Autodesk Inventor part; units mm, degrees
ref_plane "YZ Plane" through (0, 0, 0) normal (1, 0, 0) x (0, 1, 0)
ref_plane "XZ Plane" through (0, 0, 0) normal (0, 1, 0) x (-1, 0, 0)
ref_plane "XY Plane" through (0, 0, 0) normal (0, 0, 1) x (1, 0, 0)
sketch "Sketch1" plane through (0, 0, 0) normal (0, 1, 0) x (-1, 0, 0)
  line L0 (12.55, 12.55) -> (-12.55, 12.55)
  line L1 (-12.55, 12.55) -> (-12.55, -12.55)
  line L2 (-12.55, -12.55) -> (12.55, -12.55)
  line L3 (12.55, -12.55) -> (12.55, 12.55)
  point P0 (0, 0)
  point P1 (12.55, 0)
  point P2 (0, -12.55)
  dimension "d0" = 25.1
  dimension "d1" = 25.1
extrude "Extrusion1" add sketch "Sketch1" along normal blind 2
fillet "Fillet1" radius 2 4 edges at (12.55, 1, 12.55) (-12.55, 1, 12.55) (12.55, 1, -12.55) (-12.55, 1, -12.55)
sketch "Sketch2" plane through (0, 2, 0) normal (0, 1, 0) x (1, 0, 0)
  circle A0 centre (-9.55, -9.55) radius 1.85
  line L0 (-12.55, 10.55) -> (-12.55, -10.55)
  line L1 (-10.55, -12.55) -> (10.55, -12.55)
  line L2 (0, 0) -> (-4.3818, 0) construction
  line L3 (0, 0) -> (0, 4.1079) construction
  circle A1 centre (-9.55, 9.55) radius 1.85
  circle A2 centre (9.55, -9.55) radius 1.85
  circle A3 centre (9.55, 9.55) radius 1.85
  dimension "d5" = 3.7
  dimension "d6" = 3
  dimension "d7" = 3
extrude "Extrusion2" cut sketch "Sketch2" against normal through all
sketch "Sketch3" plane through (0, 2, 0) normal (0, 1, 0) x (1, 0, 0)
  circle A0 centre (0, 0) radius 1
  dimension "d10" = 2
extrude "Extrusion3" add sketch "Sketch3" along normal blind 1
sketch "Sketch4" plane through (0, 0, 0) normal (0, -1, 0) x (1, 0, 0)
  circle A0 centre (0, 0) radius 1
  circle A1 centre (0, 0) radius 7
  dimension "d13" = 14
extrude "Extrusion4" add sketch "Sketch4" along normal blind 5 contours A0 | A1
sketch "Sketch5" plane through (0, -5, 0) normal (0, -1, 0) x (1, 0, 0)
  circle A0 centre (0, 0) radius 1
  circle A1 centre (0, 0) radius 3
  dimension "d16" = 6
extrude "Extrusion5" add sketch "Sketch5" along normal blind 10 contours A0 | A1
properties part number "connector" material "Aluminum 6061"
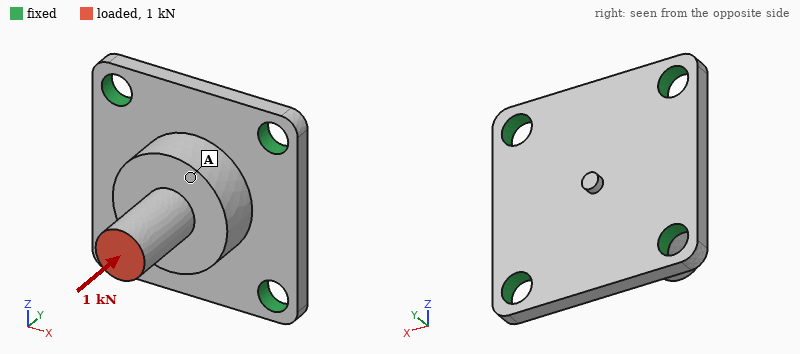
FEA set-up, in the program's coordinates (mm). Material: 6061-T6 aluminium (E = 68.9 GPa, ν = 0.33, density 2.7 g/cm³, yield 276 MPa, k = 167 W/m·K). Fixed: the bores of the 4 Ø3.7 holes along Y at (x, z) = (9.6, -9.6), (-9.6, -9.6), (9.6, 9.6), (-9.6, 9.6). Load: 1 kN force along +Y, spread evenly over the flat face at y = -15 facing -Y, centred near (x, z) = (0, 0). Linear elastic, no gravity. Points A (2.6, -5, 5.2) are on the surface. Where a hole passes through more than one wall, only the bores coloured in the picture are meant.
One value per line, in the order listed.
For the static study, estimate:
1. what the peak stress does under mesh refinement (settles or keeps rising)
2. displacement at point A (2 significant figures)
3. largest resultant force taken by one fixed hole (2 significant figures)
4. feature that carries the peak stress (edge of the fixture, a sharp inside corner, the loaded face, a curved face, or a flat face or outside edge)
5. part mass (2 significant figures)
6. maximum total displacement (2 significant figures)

keeps rising
16 µm
270 N
edge of the fixture
6.0 g
23 µm
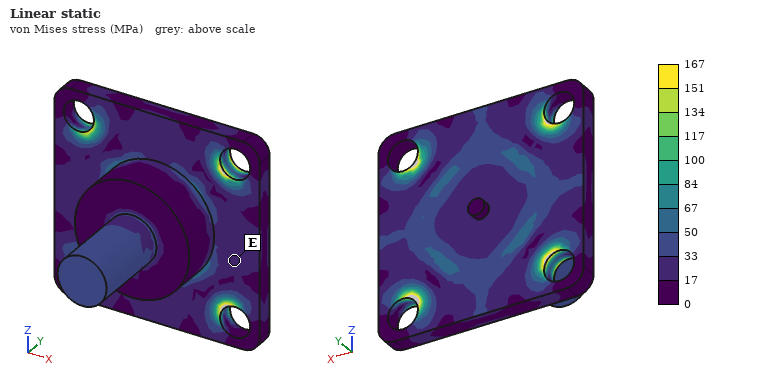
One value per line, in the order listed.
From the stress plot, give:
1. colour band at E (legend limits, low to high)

17 to 33 MPa
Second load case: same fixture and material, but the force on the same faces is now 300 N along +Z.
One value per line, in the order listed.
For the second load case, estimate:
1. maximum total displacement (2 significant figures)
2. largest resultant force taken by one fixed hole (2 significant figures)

64 µm
180 N
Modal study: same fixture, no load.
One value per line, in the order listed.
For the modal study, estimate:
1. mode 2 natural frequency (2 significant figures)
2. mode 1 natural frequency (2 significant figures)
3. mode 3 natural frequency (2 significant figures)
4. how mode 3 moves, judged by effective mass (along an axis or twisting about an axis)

18 kHz
18 kHz
19 kHz
along Y
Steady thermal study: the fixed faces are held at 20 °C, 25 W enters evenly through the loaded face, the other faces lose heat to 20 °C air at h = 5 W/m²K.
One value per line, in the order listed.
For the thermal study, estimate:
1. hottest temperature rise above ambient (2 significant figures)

77 K
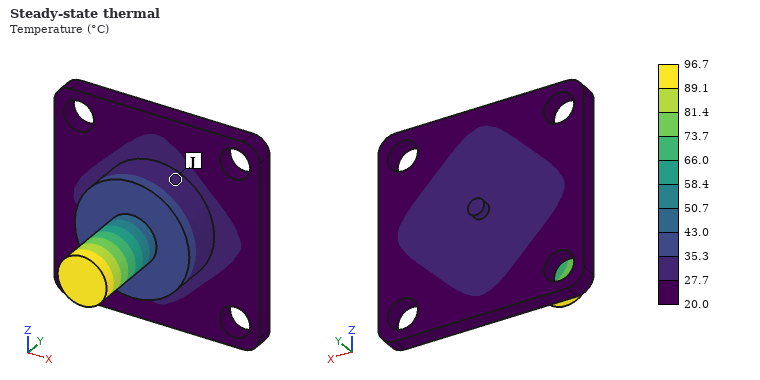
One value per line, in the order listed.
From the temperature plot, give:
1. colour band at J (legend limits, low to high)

27.7 to 35.3 °C
